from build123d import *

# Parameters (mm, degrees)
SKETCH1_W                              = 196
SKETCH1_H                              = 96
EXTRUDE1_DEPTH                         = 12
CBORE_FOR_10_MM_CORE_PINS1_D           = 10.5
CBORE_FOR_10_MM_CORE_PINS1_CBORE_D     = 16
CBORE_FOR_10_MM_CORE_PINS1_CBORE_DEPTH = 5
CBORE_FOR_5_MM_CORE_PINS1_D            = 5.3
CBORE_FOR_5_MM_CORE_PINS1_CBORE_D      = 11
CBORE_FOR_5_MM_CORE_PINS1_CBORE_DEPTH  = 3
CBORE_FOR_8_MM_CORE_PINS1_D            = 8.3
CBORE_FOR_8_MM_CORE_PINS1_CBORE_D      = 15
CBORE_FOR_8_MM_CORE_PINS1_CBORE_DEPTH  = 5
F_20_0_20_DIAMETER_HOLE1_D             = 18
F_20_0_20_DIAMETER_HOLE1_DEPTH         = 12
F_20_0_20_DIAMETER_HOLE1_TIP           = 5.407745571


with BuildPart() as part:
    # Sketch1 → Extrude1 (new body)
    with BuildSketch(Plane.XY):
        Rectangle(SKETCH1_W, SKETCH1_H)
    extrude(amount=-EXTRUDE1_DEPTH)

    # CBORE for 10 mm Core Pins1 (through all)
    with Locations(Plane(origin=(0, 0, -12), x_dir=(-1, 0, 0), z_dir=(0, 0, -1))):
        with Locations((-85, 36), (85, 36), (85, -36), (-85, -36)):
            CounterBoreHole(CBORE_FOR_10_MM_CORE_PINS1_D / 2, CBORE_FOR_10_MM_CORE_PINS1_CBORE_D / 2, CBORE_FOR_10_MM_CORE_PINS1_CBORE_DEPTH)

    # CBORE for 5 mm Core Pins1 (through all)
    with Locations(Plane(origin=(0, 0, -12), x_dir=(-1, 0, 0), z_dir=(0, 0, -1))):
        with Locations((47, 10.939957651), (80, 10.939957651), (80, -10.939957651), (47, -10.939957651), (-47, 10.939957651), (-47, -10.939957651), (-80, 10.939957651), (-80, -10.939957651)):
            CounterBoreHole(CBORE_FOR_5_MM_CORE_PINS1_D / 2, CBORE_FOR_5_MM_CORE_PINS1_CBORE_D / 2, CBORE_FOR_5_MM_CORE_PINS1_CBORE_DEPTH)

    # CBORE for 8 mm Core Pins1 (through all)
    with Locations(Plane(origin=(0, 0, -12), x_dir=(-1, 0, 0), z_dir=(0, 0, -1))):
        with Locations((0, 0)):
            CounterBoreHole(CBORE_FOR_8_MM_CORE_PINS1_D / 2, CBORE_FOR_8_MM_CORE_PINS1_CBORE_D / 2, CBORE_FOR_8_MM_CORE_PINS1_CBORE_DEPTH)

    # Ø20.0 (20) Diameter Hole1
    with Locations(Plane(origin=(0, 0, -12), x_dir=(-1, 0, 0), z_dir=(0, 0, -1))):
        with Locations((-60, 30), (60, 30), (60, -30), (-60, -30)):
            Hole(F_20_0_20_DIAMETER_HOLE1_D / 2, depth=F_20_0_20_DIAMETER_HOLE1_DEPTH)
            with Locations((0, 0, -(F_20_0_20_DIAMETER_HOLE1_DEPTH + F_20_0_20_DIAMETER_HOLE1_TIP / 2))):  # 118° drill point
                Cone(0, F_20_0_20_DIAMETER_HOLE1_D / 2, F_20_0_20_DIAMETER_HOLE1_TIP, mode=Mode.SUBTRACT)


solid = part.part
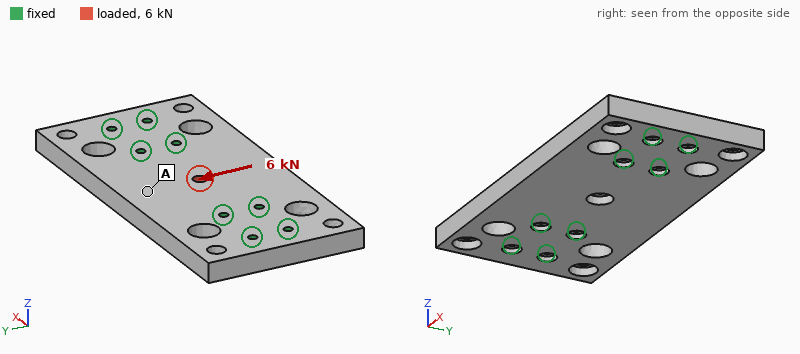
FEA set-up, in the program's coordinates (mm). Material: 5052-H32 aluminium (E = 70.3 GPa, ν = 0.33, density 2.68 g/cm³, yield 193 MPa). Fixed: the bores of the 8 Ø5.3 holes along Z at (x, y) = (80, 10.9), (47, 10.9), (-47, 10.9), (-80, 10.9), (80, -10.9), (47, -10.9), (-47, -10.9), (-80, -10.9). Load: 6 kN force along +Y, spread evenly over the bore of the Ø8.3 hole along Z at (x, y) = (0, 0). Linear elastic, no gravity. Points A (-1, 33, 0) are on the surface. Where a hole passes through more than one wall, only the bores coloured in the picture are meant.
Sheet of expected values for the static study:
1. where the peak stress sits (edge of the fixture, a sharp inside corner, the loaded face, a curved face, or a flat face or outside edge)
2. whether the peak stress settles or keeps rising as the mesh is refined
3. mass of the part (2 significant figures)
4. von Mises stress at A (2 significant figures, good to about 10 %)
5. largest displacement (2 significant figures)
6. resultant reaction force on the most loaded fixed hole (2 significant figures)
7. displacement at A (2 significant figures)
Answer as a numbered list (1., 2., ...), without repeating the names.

1. a sharp inside corner
2. keeps rising
3. 540 g
4. 3.6 MPa
5. 12 µm
6. 1.6 kN
7. 7.8 µm
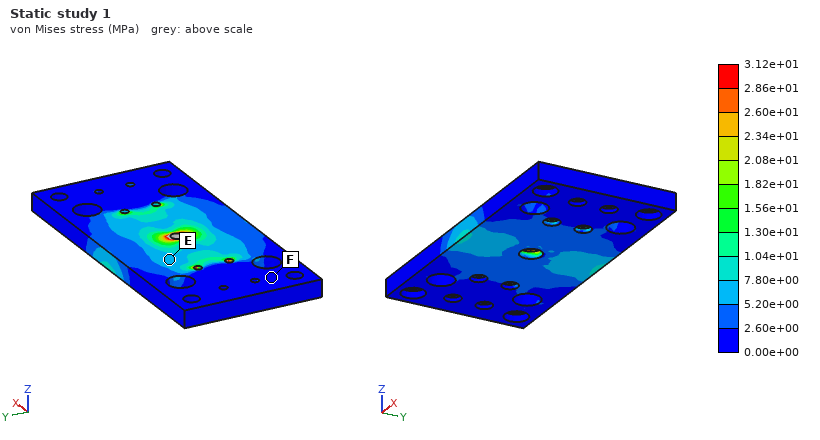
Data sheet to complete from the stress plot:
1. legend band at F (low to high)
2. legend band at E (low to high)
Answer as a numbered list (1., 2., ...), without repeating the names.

1. 0.00e+00 to 2.60e+00 MPa
2. 5.20e+00 to 7.80e+00 MPa
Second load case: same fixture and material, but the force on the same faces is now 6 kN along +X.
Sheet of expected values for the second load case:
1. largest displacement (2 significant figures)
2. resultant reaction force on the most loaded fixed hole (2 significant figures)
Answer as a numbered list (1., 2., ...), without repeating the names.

1. 7.8 µm
2. 1.3 kN
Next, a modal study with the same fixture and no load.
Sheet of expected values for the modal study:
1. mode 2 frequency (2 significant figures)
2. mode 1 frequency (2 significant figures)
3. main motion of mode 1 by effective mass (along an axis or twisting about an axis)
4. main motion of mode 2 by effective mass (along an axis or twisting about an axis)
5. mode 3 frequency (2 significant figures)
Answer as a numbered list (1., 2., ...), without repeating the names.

1. 4100 Hz
2. 3700 Hz
3. twisting about X
4. along Z
5. 6000 Hz
